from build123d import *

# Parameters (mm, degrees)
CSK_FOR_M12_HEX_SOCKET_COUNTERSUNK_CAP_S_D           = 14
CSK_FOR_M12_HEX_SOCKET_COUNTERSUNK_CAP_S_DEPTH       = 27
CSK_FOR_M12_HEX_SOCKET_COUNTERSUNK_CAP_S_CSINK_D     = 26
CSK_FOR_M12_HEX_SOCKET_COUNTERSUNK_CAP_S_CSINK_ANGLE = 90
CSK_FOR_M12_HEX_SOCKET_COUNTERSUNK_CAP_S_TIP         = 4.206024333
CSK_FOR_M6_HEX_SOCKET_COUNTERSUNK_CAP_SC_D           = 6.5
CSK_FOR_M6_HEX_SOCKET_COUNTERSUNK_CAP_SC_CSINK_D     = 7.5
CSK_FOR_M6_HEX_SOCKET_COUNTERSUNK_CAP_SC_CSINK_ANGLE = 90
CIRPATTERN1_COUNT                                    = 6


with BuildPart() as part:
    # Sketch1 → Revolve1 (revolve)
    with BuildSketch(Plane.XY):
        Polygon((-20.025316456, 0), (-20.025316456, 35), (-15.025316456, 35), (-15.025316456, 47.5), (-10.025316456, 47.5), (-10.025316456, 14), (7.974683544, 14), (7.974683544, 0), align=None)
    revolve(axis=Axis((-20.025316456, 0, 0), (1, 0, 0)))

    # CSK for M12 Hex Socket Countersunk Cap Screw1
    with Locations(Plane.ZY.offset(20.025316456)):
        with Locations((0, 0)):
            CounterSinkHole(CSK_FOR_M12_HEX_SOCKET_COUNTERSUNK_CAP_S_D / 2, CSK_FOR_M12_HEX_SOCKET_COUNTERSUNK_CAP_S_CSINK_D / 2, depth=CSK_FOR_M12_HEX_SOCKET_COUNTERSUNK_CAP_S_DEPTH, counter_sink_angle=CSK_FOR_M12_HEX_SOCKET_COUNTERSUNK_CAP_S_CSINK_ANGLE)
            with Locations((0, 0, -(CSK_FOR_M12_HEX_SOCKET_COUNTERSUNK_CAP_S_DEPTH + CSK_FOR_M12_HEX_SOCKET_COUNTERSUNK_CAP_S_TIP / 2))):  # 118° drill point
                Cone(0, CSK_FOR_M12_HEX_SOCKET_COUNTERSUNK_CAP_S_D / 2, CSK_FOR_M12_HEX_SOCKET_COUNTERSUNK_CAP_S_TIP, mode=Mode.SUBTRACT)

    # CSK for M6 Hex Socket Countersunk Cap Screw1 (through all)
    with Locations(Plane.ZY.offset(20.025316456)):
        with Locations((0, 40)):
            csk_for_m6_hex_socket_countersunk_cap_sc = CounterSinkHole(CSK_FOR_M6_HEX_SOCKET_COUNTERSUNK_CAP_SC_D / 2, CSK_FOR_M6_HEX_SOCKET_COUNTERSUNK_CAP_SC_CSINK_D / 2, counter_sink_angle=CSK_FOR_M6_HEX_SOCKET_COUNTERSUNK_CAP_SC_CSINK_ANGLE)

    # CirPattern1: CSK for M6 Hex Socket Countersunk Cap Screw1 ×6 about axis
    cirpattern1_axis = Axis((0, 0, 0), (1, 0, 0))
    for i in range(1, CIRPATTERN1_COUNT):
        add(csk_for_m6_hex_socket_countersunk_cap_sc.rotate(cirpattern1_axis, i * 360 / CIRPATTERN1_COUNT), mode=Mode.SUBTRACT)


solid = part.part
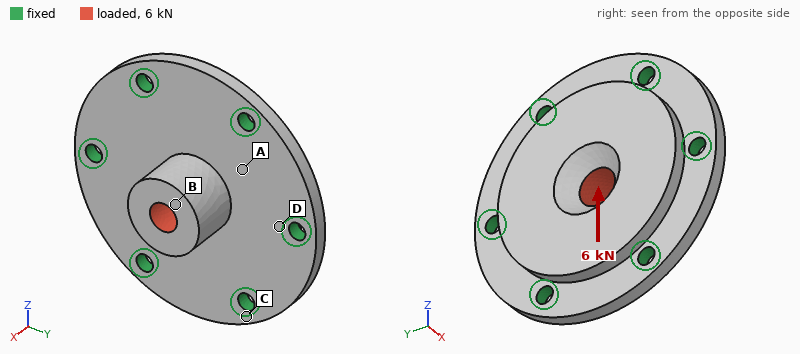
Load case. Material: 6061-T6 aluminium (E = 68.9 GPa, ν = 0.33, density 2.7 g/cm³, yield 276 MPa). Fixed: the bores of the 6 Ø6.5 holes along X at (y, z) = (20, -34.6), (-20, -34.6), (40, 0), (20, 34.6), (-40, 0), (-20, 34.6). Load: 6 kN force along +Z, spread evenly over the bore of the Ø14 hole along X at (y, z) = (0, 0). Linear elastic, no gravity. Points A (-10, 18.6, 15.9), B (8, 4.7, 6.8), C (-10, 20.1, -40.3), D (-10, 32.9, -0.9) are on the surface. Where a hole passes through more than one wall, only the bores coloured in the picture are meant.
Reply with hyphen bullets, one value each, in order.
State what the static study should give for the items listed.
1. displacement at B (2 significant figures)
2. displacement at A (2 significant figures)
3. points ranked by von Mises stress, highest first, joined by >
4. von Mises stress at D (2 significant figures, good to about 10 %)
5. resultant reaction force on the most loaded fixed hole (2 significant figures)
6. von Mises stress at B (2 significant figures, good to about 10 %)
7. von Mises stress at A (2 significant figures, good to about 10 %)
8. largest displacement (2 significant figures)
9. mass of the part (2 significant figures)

- 30 µm
- 5.9 µm
- A > D > B > C
- 12 MPa
- 1.3 kN
- 8.8 MPa
- 18 MPa
- 33 µm
- 160 g
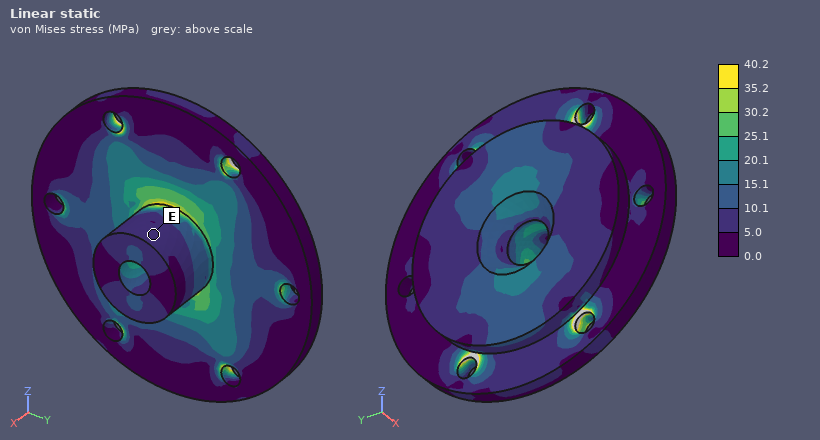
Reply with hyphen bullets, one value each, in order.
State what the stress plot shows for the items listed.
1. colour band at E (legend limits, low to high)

- 5.0 to 10.1 MPa
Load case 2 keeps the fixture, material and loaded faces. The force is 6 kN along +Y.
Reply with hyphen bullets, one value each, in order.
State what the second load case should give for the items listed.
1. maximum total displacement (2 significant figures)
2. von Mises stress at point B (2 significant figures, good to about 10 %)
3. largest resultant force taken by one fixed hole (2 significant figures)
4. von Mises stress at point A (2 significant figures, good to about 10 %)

- 33 µm
- 6.0 MPa
- 1.4 kN
- 13 MPa
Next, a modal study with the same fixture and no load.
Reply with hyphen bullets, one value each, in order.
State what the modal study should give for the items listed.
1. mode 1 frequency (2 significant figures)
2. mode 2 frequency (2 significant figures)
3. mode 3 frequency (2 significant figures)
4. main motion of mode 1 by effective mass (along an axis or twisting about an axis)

- 8100 Hz
- 12 kHz
- 12 kHz
- along X
